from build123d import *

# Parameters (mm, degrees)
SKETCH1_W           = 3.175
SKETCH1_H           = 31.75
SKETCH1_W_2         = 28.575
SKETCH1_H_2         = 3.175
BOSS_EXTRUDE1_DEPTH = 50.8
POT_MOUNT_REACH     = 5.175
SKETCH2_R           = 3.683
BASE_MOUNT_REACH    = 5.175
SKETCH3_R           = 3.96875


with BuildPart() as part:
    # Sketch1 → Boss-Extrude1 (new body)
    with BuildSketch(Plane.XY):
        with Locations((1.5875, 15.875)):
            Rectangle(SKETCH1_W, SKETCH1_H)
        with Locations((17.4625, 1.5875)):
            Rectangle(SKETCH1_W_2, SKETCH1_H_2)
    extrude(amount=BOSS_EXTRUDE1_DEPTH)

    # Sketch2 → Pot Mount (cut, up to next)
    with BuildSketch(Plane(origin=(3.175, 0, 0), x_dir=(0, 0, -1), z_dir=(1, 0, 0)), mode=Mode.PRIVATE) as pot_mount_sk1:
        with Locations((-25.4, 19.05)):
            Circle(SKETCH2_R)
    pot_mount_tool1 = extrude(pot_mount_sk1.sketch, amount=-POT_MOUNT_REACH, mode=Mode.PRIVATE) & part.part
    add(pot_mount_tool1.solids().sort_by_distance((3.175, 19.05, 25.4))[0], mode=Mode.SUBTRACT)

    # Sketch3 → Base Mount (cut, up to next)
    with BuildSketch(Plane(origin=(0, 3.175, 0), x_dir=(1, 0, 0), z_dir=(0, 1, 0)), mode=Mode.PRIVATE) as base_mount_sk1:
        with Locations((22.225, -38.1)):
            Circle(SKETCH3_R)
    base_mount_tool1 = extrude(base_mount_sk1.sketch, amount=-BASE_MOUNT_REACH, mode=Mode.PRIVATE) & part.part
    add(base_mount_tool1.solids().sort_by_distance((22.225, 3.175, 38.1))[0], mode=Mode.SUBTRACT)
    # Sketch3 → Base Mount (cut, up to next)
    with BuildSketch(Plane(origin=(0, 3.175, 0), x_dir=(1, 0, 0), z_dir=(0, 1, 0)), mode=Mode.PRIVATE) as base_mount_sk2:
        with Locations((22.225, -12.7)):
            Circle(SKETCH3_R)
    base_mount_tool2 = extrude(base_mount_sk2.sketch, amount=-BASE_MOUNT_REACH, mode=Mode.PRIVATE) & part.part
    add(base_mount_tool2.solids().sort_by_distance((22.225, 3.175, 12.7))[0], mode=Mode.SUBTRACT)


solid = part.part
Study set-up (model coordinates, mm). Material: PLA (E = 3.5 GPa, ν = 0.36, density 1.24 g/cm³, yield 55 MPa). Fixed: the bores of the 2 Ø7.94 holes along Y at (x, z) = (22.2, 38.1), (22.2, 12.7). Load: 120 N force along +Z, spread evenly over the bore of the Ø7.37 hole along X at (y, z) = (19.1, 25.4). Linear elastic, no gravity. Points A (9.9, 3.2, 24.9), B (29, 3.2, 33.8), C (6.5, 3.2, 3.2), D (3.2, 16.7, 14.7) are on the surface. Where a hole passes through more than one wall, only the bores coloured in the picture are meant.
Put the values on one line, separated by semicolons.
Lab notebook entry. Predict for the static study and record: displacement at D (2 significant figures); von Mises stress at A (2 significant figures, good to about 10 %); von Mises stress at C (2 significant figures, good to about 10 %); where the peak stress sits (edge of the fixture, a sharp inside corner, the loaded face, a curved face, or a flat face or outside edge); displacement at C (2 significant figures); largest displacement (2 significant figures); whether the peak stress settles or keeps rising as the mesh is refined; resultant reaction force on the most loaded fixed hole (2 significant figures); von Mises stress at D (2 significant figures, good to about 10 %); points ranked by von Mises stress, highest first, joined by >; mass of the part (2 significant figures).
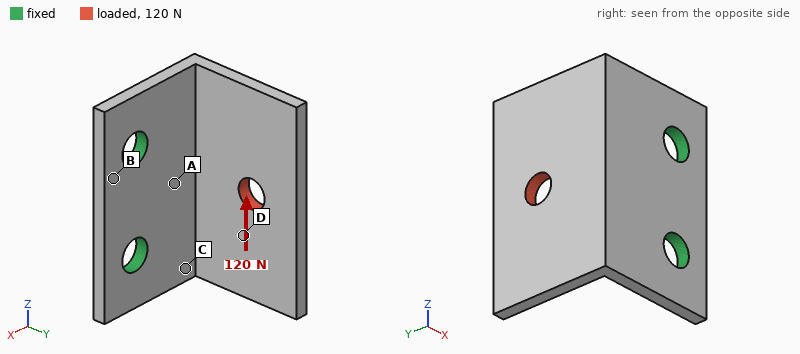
0.36 mm; 10 MPa; 7.0 MPa; edge of the fixture; 0.28 mm; 0.78 mm; keeps rising; 110 N; 4.0 MPa; A > C > D > B; 12 g
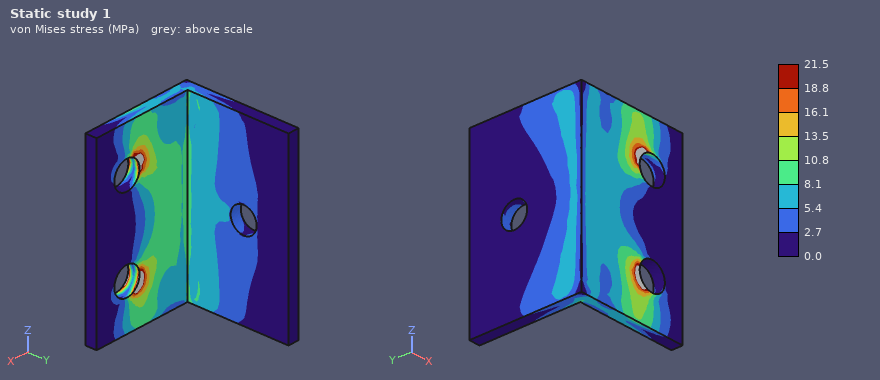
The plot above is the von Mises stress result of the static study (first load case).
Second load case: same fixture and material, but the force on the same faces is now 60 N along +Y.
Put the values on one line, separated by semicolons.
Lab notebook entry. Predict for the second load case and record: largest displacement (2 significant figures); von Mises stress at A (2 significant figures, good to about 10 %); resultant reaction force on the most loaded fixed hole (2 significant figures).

0.66 mm; 5.2 MPa; 30 N
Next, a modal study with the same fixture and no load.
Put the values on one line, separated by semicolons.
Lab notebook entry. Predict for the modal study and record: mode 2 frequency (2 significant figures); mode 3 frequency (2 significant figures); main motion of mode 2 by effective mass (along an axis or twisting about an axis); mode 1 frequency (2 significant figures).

880 Hz; 1500 Hz; along Z; 500 Hz
